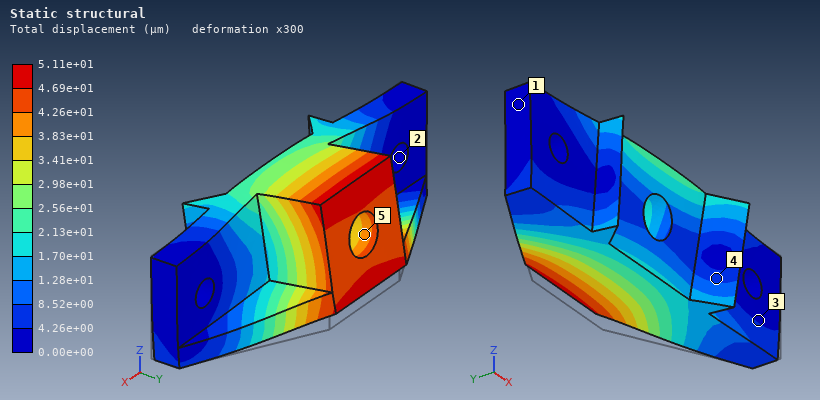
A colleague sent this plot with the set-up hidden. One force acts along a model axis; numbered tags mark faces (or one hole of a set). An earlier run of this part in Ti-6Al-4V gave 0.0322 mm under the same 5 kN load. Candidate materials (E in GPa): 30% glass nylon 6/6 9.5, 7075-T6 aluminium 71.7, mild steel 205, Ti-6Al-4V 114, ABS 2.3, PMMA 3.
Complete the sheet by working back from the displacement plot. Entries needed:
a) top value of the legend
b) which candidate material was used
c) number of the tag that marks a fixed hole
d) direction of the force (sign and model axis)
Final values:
5.11e+01 µm
7075-T6 aluminium
2
+Z
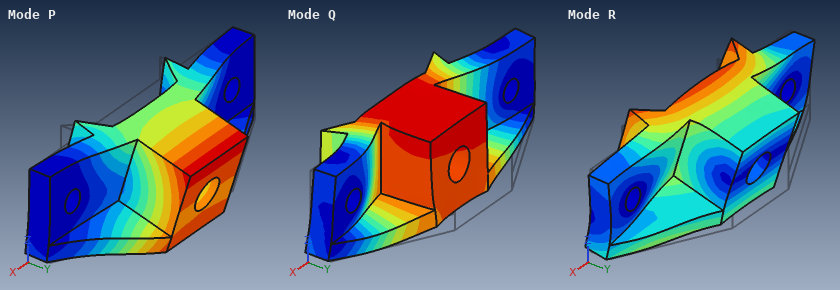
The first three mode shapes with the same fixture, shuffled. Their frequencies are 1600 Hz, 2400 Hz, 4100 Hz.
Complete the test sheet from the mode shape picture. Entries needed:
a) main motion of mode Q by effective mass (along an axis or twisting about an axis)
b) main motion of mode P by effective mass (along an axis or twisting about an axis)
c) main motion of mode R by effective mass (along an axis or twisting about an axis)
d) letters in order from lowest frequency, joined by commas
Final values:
along Y
along Z
along Z
P, Q, R
